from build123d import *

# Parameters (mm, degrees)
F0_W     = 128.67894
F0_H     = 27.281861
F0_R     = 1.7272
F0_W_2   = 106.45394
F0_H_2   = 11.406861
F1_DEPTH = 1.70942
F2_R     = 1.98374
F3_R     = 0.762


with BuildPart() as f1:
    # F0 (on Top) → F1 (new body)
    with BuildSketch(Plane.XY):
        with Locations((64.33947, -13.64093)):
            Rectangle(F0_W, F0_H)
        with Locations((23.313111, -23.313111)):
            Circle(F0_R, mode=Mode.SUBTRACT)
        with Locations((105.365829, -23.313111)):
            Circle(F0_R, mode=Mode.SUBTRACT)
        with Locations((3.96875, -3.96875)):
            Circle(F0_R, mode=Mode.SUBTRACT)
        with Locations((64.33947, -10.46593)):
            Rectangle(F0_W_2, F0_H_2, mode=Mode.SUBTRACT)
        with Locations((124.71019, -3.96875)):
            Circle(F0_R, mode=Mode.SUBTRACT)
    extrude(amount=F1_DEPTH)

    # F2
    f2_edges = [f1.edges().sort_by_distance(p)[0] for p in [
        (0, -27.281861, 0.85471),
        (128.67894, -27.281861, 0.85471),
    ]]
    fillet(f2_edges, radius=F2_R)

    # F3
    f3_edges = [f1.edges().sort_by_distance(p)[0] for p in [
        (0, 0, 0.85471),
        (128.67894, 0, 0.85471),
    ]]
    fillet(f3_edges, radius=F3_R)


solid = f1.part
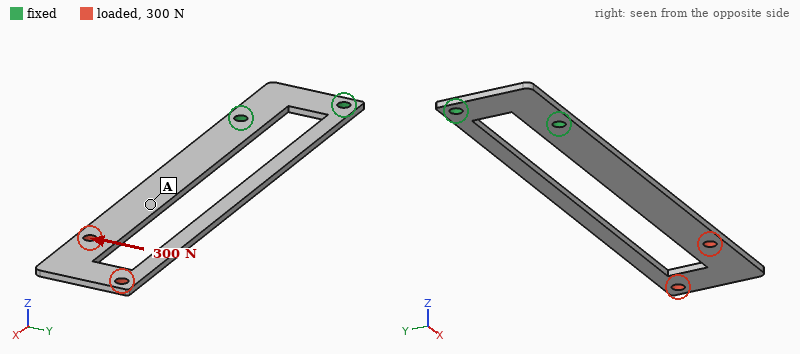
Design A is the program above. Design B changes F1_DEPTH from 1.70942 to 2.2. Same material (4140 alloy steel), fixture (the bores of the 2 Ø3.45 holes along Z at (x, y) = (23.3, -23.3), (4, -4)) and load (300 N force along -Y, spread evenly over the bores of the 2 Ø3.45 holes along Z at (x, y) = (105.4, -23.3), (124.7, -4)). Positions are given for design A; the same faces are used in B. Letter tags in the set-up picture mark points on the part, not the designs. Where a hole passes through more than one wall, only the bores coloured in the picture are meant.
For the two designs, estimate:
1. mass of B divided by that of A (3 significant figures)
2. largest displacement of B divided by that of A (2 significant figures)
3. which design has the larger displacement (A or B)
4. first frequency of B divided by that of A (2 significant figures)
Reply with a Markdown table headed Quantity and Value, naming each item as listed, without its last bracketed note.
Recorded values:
| Quantity | Value |
|---|---|
| mass of B divided by that of A | 1.29 |
| largest displacement of B divided by that of A | 0.78 |
| which design has the larger displacement | A |
| first frequency of B divided by that of A | 1.3 |
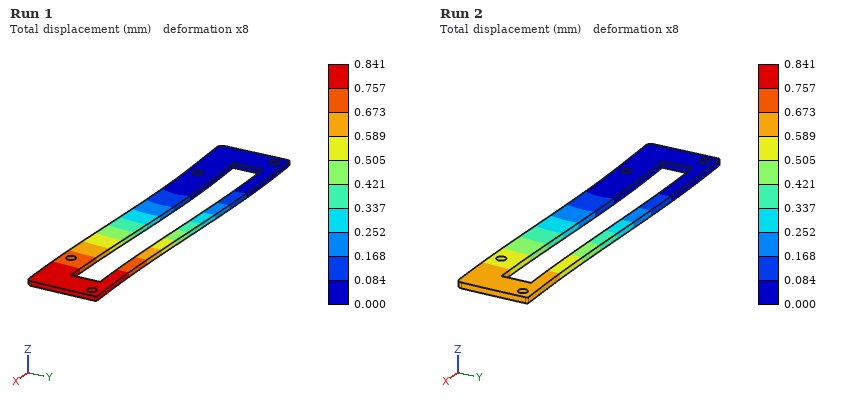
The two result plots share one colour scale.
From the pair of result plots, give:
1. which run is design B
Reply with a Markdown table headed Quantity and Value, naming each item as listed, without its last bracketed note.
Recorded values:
| Quantity | Value |
|---|---|
| which run is design B | Run 2 |
